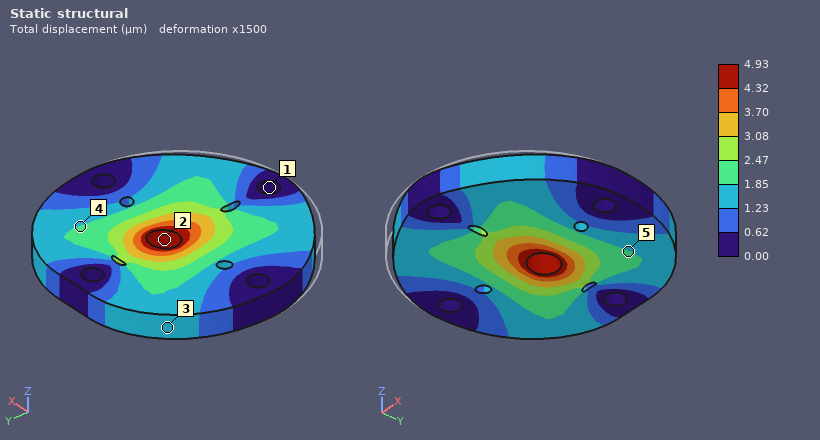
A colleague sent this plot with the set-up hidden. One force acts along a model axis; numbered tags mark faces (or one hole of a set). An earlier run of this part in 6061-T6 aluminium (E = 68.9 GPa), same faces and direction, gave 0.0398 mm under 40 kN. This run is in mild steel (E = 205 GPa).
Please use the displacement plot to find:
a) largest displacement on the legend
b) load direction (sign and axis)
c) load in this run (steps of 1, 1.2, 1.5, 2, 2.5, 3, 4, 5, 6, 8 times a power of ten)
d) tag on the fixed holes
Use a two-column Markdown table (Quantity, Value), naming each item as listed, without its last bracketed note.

| Quantity | Value |
|---|---|
| largest displacement on the legend | 4.93 µm |
| load direction | +Y |
| load in this run | 15 kN |
| tag on the fixed holes | 1 |
